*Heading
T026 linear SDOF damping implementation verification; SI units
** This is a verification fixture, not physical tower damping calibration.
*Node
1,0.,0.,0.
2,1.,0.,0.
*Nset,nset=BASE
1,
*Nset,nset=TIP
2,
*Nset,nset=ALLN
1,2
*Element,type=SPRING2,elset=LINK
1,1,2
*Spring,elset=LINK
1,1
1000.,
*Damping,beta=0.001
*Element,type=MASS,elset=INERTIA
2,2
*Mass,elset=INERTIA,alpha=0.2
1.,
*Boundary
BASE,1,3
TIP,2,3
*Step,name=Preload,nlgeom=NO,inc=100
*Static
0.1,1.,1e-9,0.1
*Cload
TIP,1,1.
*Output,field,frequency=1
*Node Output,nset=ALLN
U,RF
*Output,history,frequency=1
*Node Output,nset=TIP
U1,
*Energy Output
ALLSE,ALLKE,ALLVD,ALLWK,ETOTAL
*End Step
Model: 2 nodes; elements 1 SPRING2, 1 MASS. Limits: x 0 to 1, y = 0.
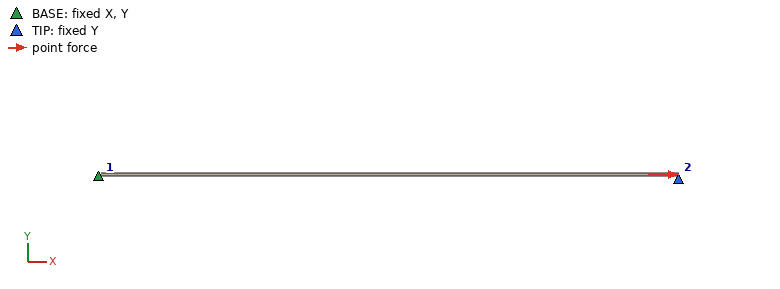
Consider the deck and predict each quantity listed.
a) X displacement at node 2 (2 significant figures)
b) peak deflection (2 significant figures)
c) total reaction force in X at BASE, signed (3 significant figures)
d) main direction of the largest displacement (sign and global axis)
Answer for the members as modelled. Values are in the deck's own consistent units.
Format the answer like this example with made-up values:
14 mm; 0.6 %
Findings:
0.0010; 0.0010; -1.00; +X
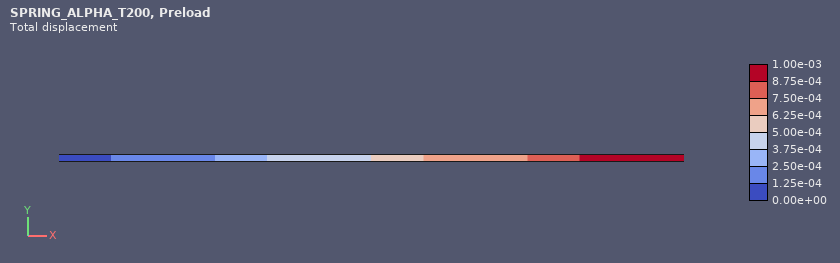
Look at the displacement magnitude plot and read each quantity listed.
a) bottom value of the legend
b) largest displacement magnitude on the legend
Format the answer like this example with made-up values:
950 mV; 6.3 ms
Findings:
0.00e+00; 1.00e-03
